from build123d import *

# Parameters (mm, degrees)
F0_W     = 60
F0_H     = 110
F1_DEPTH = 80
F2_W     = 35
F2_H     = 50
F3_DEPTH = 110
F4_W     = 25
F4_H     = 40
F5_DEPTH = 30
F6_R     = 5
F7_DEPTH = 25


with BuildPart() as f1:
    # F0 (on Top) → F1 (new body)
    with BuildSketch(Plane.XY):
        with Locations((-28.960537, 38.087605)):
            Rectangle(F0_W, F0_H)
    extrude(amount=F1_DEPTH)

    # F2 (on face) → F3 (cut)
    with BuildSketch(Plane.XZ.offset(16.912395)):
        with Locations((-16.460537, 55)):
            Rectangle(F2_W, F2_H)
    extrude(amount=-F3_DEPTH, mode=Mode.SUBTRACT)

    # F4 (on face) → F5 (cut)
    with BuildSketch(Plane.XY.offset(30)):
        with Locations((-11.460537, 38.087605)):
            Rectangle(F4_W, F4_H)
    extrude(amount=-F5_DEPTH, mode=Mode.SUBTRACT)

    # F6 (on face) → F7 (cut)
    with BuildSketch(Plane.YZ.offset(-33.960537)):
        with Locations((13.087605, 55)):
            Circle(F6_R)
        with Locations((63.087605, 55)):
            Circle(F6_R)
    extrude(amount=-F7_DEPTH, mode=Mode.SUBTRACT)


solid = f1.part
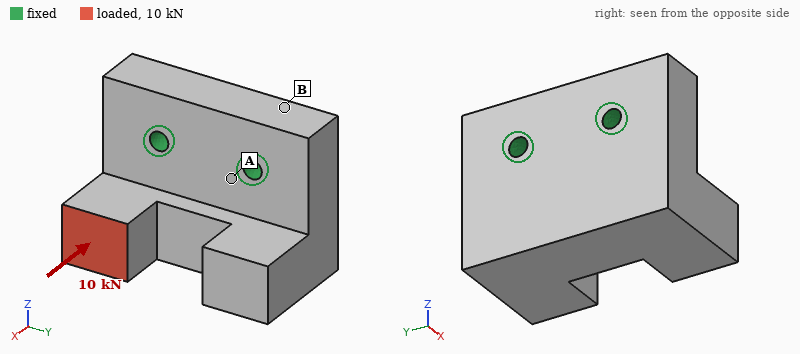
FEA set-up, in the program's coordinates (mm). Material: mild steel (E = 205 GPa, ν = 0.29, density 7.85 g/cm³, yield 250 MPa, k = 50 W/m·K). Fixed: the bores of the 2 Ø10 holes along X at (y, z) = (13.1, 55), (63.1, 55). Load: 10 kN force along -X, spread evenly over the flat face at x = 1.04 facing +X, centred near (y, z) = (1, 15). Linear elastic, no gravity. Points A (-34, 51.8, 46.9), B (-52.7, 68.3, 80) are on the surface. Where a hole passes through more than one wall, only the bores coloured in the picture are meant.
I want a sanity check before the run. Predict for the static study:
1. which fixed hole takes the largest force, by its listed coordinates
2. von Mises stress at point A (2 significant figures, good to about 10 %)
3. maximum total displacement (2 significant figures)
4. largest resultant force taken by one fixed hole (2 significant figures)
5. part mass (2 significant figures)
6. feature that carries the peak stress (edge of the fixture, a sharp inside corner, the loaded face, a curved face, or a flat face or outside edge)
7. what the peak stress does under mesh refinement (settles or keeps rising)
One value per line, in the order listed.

(13.1, 55)
24 MPa
41 µm
10 kN
2.4 kg
edge of the fixture
keeps rising
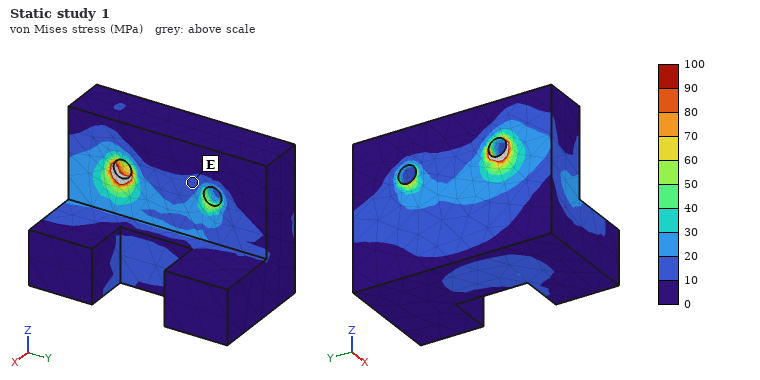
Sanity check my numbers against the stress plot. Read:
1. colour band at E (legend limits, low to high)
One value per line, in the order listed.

10 to 20 MPa
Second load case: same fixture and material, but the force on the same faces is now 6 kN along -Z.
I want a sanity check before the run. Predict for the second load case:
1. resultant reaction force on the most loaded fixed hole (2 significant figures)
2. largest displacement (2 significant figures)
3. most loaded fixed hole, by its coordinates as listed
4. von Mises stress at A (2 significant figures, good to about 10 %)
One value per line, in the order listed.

7.0 kN
46 µm
(13.1, 55)
19 MPa
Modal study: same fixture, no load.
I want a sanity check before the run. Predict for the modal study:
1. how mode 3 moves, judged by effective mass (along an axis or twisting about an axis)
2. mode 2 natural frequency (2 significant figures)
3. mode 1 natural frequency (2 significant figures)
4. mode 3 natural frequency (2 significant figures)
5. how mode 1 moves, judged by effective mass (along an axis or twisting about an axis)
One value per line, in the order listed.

along Y
4400 Hz
3200 Hz
6000 Hz
along X
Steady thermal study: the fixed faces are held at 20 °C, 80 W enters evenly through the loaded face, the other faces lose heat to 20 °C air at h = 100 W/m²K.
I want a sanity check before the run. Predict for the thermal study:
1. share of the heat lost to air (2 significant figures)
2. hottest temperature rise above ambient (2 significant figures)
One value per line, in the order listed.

49 %
70 K
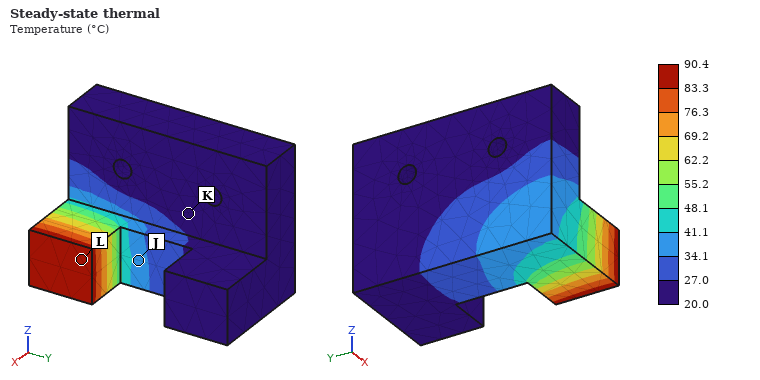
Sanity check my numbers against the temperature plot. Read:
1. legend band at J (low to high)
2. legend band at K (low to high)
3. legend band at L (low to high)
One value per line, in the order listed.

34.1 to 41.1 °C
20.0 to 27.0 °C
83.3 to 90.4 °C
